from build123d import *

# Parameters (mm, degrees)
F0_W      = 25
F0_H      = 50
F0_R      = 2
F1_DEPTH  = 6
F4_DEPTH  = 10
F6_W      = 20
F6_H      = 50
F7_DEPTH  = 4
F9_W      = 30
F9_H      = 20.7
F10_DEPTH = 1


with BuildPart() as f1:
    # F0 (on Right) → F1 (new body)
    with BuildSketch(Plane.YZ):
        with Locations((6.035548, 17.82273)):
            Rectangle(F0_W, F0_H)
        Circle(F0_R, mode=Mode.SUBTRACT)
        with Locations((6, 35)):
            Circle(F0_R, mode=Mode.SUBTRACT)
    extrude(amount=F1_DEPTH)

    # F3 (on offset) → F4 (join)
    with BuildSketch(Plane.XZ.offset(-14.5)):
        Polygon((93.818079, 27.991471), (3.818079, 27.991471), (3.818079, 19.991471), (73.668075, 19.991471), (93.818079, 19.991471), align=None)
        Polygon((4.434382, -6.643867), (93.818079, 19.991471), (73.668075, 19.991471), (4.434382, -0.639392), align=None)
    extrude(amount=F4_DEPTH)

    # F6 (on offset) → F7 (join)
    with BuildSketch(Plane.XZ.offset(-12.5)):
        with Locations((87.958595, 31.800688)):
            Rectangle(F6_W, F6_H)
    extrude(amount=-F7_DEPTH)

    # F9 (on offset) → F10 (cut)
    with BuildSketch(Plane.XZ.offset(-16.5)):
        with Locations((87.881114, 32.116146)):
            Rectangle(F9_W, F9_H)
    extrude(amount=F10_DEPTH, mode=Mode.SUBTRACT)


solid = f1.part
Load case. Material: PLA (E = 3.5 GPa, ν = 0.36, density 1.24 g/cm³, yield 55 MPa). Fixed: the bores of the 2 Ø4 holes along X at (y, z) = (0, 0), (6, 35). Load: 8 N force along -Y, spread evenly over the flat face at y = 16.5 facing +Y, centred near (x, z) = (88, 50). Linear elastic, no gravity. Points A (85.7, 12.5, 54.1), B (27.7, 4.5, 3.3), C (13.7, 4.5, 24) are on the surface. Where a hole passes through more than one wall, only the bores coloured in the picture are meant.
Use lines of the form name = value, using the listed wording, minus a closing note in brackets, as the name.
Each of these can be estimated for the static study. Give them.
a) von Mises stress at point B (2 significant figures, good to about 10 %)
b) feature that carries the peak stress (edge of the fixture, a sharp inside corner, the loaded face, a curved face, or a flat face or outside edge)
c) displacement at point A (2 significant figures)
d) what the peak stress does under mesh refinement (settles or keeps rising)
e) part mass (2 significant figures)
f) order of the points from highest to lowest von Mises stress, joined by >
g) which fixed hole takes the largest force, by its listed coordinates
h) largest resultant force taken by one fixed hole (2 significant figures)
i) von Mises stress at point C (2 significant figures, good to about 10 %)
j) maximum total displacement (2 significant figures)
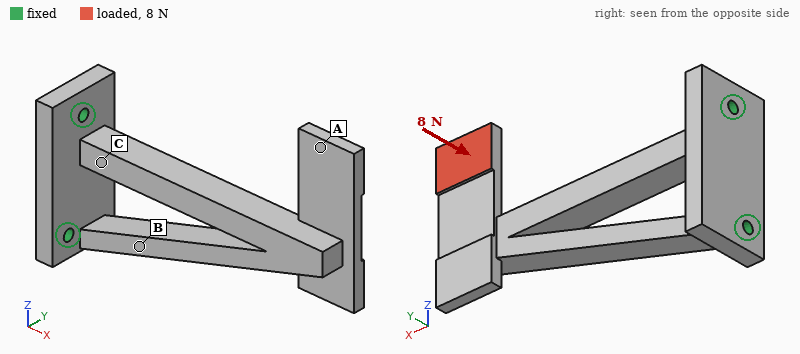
von Mises stress at point B = 1.9 MPa
feature that carries the peak stress = edge of the fixture
displacement at point A = 1.1 mm
what the peak stress does under mesh refinement = keeps rising
part mass = 28 g
order of the points from highest to lowest von Mises stress, joined by > = C > B > A
which fixed hole takes the largest force, by its listed coordinates = (6, 35)
largest resultant force taken by one fixed hole = 12 N
von Mises stress at point C = 3.4 MPa
maximum total displacement = 1.2 mm
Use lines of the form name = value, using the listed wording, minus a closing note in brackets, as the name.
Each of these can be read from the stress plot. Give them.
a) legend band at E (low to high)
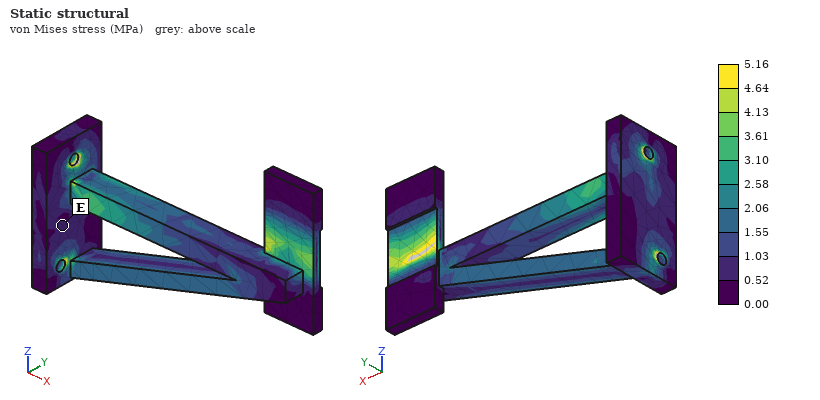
legend band at E = 0.52 to 1.03 MPa
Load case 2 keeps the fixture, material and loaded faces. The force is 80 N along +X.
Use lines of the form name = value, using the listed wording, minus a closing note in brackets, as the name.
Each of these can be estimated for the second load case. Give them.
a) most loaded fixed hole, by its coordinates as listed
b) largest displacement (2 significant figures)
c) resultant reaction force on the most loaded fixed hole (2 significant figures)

most loaded fixed hole, by its coordinates as listed = (6, 35)
largest displacement = 1.4 mm
resultant reaction force on the most loaded fixed hole = 120 N
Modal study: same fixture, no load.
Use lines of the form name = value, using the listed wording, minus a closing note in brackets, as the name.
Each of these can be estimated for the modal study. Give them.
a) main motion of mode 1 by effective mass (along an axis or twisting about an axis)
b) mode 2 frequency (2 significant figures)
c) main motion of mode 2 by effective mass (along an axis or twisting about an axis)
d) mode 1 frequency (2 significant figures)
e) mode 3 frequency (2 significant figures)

main motion of mode 1 by effective mass = along Y
mode 2 frequency = 540 Hz
main motion of mode 2 by effective mass = along Z
mode 1 frequency = 200 Hz
mode 3 frequency = 590 Hz
